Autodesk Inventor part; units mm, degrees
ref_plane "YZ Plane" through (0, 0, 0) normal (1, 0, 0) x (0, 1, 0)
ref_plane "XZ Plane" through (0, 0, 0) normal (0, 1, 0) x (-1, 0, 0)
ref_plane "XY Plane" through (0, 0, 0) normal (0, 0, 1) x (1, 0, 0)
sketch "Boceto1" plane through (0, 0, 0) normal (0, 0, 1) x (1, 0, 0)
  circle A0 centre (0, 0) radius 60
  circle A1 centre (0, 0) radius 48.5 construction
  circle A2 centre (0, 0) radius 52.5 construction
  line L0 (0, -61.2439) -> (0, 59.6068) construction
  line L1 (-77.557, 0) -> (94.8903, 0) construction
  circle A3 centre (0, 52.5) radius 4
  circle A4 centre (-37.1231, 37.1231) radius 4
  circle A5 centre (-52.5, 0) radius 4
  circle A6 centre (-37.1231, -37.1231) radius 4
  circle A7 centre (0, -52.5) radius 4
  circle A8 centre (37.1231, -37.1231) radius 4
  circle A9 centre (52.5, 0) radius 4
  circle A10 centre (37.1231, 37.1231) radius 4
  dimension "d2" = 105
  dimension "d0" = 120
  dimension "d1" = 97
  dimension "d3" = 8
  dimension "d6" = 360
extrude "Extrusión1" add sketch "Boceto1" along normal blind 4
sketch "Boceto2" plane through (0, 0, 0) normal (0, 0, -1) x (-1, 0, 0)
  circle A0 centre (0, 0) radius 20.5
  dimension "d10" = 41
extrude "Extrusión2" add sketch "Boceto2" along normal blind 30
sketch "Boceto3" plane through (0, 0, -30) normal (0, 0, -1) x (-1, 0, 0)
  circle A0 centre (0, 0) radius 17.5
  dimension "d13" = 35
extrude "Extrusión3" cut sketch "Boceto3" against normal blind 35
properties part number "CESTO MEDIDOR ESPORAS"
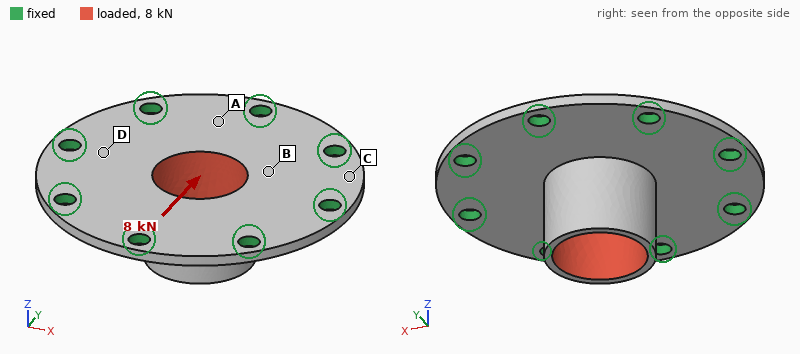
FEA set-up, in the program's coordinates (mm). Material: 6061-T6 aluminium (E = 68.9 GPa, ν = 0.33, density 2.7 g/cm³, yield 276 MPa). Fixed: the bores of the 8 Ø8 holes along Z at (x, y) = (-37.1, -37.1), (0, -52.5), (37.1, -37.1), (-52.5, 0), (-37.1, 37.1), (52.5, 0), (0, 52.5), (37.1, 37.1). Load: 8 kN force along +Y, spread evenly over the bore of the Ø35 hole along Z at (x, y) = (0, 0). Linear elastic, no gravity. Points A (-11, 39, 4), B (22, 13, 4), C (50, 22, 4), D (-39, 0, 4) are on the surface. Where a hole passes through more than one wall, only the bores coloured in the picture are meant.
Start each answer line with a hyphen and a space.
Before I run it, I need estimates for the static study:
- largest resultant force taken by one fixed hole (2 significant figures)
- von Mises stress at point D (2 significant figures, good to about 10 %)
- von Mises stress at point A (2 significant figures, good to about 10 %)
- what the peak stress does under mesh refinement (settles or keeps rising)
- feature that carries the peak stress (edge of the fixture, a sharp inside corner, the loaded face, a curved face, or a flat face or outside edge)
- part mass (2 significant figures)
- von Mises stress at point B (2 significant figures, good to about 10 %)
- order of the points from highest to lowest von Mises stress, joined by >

- 1.9 kN
- 35 MPa
- 56 MPa
- keeps rising
- edge of the fixture
- 140 g
- 77 MPa
- B > A > D > C
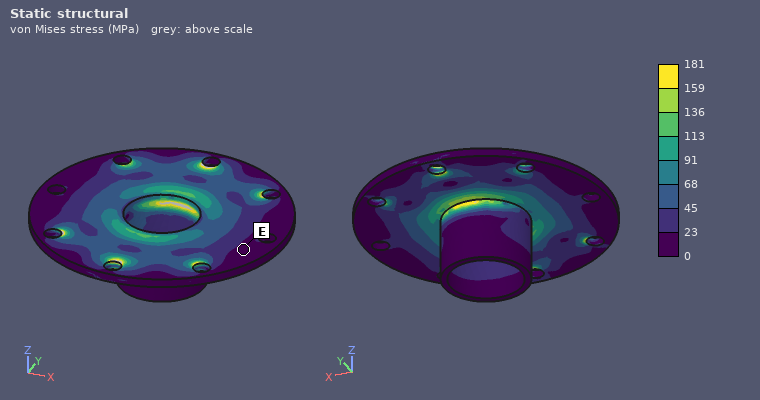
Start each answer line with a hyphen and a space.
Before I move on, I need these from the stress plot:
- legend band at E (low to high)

- 0 to 23 MPa
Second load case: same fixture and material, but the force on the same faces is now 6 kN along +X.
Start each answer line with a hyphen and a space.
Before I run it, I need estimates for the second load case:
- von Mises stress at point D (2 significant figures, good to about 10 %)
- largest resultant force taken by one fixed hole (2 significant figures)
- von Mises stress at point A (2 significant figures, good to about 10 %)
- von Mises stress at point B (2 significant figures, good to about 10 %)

- 37 MPa
- 1.4 kN
- 23 MPa
- 69 MPa
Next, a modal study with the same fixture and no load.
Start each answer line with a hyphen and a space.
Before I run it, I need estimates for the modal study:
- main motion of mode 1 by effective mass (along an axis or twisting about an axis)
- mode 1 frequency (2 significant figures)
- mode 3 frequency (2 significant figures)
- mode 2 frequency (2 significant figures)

- along Z
- 3300 Hz
- 4000 Hz
- 4000 Hz
